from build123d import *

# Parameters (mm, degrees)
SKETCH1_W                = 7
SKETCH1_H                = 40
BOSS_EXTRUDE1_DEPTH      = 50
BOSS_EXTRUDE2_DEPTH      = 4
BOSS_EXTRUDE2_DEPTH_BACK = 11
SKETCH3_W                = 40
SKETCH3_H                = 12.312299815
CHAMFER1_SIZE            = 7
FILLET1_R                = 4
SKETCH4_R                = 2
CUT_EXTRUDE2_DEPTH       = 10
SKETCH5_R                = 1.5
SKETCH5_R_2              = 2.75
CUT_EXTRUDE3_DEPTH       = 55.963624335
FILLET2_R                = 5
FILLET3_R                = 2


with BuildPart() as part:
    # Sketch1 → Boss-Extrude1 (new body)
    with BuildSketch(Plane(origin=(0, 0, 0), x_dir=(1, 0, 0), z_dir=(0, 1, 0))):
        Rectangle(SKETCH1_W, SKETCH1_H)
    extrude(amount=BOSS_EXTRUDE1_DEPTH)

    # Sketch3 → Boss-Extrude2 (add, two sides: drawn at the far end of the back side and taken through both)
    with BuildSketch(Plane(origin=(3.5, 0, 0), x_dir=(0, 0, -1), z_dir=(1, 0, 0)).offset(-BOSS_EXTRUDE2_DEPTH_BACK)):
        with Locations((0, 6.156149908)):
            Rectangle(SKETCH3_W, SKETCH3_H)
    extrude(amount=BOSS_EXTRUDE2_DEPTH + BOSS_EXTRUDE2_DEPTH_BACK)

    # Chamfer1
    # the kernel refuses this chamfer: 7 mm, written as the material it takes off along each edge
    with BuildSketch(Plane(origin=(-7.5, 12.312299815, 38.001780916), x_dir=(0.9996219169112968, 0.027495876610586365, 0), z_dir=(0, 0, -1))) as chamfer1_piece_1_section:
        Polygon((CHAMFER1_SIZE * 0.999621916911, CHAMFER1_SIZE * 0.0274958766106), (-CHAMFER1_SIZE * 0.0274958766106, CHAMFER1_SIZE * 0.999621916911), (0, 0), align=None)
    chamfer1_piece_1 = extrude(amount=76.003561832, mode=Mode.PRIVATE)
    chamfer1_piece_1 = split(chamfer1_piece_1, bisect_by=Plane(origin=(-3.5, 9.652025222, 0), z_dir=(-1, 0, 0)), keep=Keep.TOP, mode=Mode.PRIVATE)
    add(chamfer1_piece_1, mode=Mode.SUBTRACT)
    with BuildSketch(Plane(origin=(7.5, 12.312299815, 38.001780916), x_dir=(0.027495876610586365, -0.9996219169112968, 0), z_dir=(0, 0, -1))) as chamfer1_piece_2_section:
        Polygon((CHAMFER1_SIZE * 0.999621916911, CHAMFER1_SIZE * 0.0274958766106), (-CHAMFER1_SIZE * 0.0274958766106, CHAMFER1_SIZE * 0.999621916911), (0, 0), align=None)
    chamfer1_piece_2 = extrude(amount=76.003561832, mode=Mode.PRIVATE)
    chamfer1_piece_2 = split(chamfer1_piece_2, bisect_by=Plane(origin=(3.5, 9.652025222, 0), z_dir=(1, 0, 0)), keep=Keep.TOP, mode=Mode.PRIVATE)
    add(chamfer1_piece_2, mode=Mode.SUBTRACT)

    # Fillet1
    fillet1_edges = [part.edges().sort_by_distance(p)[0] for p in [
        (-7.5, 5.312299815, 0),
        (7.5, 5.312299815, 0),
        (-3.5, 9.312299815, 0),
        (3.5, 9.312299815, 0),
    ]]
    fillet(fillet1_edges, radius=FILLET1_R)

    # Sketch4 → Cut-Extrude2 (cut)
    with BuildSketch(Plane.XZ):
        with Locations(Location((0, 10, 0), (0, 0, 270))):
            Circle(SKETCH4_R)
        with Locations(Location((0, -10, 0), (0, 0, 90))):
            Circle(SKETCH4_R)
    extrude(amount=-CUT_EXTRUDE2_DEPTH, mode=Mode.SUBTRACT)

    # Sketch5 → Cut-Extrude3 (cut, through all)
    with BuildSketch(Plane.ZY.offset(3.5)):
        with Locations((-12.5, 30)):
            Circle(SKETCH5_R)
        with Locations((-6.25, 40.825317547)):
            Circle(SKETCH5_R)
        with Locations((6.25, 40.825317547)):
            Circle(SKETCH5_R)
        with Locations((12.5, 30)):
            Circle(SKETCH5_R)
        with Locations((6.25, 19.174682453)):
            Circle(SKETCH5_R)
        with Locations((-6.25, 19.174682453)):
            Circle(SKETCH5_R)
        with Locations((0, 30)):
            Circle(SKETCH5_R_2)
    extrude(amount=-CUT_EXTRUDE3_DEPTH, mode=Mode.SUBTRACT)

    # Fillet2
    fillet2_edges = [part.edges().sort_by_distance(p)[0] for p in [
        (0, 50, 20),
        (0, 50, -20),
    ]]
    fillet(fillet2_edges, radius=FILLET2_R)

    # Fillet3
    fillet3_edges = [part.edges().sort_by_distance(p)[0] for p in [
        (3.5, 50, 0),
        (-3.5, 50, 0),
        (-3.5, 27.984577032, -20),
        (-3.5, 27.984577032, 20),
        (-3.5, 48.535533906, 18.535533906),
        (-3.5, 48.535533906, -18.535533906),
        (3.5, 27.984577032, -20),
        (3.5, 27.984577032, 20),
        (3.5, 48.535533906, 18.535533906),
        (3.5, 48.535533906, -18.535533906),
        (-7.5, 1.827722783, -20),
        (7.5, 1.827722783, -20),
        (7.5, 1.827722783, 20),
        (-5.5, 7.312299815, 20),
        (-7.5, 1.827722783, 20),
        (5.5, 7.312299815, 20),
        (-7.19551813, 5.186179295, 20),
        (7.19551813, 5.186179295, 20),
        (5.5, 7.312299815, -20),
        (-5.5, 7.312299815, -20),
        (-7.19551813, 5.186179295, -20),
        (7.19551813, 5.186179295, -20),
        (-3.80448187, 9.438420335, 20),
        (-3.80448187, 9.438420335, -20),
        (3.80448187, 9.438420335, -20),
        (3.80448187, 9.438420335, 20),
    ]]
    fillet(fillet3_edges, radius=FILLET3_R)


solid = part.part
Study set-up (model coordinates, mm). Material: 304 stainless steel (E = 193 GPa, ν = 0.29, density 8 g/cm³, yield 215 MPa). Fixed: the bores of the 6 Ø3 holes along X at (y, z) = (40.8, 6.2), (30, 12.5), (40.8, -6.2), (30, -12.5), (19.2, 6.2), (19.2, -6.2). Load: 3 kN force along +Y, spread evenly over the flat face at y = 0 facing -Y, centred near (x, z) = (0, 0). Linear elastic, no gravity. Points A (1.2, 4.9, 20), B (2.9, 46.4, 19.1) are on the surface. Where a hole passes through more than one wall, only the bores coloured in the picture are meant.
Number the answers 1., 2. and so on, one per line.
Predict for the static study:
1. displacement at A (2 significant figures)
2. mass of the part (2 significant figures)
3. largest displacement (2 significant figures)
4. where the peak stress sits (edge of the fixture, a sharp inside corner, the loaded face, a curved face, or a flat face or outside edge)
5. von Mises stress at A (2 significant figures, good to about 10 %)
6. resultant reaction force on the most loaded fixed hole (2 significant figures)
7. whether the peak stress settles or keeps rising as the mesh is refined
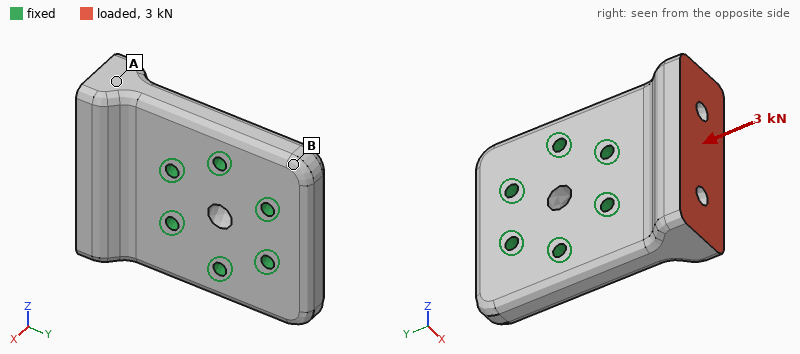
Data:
1. 1.1 µm
2. 120 g
3. 1.3 µm
4. edge of the fixture
5. 7.2 MPa
6. 1.0 kN
7. keeps rising
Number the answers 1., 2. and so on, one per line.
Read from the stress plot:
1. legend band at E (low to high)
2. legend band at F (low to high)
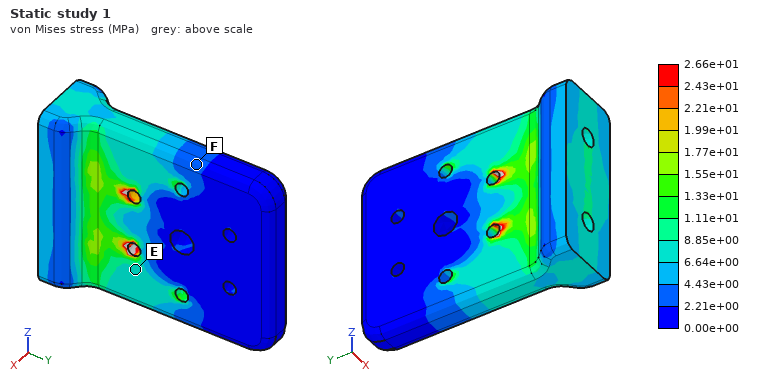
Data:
1. 6.64e+00 to 8.85e+00 MPa
2. 2.21e+00 to 4.43e+00 MPa
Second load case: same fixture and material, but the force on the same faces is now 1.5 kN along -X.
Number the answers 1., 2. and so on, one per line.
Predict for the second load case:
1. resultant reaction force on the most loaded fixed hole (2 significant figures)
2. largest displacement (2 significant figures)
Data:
1. 1.1 kN
2. 23 µm
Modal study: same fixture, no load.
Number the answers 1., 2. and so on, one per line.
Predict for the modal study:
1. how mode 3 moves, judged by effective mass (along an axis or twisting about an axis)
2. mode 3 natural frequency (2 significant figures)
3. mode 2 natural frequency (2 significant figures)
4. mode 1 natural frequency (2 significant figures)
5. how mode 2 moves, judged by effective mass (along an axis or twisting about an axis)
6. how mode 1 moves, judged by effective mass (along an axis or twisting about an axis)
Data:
1. along Z
2. 20 kHz
3. 12 kHz
4. 8700 Hz
5. twisting about Y
6. along X
